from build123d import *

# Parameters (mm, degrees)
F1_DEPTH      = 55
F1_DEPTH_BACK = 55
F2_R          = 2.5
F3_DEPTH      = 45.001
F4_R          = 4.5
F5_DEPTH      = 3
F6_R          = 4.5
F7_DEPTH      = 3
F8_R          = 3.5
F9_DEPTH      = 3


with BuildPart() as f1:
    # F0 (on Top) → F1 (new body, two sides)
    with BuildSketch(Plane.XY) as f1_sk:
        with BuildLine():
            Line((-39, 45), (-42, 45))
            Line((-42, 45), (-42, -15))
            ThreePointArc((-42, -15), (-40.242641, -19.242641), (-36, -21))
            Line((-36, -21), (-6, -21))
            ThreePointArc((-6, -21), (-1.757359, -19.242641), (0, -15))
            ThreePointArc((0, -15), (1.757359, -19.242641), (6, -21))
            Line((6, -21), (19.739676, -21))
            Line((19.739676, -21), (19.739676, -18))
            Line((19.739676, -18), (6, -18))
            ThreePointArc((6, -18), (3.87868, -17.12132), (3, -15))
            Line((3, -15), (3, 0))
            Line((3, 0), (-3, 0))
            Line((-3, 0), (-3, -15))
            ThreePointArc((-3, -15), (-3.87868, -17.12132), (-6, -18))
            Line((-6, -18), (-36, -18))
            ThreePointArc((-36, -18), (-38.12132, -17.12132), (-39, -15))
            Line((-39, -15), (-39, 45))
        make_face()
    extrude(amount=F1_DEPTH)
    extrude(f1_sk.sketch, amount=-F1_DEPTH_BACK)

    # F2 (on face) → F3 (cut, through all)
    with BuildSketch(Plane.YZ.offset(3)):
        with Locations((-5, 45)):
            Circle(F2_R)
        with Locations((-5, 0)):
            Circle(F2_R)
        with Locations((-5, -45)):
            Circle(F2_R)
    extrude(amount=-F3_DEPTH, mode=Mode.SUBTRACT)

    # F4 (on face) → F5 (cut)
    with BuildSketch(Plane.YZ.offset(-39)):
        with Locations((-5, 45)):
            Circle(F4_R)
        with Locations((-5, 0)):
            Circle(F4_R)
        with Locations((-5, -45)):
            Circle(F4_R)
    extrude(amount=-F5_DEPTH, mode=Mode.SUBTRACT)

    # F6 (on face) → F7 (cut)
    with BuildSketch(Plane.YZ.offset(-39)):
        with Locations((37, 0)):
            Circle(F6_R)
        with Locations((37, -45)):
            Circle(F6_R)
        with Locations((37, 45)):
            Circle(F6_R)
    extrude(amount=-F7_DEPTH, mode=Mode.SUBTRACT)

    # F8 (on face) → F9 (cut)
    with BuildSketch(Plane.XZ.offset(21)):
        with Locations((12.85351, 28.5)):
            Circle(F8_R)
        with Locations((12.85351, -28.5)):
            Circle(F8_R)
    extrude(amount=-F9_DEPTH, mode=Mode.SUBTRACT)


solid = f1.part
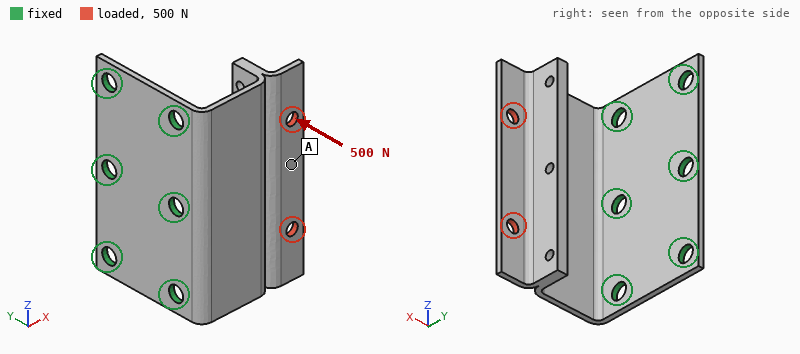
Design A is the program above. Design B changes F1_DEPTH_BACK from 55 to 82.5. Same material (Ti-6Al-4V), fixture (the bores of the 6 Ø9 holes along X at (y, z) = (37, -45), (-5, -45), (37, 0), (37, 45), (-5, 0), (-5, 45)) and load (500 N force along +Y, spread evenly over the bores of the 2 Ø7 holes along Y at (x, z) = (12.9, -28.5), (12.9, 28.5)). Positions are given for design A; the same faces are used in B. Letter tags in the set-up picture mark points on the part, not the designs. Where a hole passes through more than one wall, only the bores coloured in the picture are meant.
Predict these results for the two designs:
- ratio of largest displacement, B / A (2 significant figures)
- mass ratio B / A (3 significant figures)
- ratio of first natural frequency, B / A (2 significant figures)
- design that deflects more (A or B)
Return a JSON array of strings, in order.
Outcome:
["0.88", "1.26", "0.98", "A"]
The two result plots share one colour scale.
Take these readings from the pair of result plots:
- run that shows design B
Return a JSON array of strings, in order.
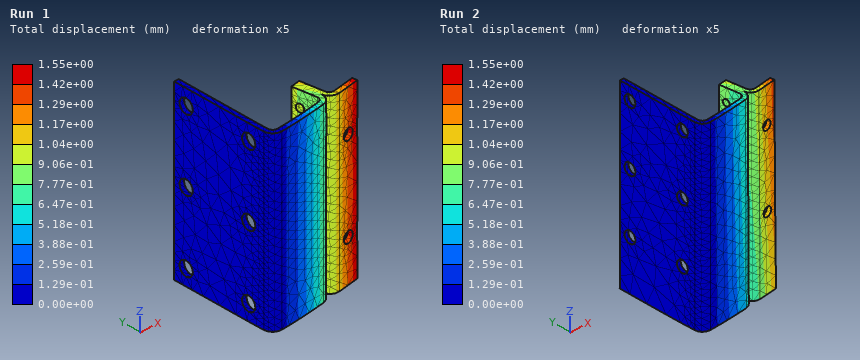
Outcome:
["Run 2"]
